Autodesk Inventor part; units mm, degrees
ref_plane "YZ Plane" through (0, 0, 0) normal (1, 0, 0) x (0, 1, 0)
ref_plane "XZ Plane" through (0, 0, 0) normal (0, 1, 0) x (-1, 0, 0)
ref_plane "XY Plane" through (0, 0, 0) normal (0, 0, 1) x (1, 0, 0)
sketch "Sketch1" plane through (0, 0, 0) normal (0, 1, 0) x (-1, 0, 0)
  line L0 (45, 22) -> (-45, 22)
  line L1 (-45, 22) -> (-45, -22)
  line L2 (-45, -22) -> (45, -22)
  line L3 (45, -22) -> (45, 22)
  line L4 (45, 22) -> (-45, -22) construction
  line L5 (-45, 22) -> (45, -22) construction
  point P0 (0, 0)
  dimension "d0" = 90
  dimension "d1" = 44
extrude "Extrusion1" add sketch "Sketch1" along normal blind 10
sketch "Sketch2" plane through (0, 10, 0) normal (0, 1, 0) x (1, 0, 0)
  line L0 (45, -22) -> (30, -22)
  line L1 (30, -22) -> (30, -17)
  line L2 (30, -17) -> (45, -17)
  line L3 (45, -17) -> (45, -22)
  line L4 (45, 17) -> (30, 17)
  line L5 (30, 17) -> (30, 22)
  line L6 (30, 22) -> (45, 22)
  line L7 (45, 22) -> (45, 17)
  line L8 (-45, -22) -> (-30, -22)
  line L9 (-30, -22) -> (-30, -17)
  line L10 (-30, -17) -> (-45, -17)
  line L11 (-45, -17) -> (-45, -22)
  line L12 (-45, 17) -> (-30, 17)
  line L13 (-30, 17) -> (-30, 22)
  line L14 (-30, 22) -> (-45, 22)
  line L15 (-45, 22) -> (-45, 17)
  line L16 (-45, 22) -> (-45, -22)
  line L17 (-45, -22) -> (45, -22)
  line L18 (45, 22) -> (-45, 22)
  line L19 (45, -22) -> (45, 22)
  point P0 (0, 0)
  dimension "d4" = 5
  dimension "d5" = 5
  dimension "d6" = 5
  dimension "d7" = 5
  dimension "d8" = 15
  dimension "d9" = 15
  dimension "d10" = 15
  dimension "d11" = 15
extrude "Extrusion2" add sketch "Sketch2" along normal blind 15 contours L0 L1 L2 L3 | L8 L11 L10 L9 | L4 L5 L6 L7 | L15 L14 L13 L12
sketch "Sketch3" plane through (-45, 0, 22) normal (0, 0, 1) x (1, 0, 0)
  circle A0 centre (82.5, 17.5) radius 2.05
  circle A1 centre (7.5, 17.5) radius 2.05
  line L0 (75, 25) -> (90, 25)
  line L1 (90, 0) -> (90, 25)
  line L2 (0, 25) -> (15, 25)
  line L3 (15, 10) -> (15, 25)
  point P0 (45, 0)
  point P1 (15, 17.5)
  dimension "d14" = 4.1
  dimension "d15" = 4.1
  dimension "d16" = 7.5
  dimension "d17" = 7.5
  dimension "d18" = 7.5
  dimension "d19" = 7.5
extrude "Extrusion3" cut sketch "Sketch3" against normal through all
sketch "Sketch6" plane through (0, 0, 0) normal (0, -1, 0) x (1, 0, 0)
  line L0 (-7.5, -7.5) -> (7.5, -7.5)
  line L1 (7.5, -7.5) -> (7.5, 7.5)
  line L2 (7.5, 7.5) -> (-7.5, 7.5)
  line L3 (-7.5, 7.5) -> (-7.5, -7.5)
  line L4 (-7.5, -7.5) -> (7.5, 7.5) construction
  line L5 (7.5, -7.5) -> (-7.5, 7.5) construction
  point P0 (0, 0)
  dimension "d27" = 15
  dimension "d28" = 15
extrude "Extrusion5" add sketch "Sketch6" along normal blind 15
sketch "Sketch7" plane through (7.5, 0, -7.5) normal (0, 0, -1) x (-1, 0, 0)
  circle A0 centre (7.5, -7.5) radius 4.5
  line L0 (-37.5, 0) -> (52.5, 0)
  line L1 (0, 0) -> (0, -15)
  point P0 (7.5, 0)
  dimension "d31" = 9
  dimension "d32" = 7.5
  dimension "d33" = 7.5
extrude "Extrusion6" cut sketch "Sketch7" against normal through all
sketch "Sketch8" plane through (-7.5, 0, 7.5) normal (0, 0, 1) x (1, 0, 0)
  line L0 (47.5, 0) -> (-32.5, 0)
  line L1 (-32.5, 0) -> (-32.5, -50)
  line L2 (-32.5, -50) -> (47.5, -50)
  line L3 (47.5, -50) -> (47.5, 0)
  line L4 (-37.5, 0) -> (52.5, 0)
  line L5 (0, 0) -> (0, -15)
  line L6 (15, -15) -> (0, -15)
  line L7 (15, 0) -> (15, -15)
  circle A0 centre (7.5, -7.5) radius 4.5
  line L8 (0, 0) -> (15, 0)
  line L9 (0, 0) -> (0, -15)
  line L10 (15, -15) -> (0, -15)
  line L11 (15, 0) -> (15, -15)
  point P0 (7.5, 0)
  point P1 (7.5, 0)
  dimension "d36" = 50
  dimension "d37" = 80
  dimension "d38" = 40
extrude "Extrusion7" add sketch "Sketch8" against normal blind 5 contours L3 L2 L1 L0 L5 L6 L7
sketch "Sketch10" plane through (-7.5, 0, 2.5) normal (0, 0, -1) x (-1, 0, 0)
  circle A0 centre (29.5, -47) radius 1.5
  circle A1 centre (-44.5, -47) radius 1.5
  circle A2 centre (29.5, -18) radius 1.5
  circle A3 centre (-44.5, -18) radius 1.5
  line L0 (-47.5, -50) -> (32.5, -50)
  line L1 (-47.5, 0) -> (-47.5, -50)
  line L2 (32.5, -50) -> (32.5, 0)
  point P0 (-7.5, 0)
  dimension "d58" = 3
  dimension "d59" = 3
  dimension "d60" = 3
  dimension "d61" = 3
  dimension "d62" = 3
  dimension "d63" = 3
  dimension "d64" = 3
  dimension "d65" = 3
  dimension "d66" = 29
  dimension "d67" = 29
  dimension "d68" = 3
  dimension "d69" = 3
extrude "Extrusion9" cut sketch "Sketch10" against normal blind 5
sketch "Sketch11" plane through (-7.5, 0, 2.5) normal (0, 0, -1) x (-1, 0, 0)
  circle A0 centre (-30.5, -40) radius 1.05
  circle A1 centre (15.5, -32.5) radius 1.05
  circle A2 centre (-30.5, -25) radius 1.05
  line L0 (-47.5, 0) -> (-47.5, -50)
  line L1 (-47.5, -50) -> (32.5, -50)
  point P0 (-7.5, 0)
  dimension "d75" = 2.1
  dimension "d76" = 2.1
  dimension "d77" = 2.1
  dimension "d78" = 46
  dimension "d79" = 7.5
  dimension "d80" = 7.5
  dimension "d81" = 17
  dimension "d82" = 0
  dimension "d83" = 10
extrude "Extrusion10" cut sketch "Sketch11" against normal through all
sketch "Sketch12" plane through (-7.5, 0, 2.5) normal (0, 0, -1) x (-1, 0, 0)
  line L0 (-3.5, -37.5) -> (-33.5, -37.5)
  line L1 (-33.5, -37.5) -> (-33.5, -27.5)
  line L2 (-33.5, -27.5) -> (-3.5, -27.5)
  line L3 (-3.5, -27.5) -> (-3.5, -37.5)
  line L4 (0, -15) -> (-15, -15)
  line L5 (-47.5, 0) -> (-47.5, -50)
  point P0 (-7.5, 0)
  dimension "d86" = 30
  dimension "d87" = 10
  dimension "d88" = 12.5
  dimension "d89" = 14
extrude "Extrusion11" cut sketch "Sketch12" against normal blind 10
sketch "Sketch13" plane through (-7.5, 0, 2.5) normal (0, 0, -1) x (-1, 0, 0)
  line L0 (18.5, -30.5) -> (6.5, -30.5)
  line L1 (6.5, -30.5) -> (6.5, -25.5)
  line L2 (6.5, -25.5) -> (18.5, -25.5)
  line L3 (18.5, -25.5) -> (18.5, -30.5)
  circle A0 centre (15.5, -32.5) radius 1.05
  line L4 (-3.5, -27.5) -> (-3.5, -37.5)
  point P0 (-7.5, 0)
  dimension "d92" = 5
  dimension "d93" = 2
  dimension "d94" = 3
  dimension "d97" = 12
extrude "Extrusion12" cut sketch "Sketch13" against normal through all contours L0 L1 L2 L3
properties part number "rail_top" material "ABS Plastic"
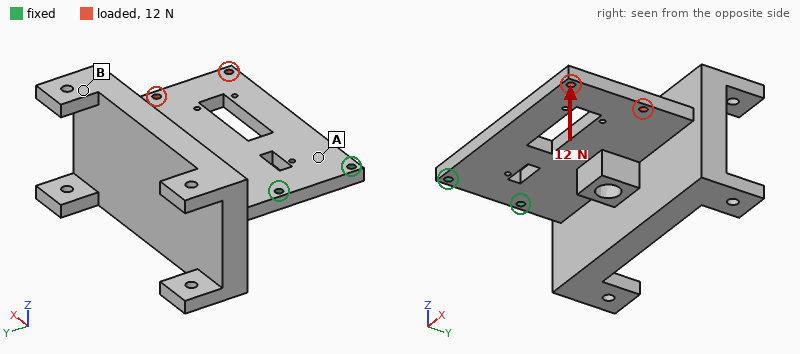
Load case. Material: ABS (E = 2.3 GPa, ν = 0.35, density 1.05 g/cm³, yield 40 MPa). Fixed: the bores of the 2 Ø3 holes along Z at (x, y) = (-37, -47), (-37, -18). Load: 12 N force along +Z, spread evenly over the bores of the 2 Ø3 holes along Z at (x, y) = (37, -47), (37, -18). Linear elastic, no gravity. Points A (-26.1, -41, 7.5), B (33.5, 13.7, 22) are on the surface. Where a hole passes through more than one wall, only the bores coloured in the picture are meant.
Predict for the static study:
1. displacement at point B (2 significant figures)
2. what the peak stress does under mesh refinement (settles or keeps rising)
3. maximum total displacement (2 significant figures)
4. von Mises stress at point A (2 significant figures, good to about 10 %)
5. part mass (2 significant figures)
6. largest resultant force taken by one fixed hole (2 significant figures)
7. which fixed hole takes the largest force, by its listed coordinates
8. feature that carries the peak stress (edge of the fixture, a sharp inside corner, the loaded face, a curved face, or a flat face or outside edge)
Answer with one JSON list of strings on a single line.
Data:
["1.0 mm", "keeps rising", "1.3 mm", "3.0 MPa", "66 g", "9.0 N", "(-37, -18)", "edge of the fixture"]
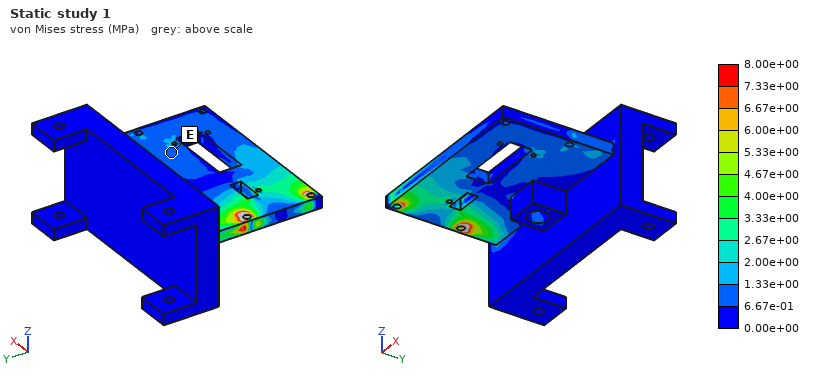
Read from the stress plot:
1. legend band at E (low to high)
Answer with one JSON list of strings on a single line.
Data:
["6.67e-01 to 1.33e+00 MPa"]
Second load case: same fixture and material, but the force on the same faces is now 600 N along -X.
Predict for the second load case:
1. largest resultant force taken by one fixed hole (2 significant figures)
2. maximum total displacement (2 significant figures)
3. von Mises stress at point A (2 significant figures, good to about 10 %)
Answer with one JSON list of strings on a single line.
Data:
["310 N", "0.24 mm", "3.5 MPa"]
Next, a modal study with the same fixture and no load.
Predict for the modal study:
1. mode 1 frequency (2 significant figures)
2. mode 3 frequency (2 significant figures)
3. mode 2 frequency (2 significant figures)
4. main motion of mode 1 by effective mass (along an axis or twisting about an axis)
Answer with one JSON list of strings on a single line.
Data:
["93 Hz", "490 Hz", "260 Hz", "along Z"]
